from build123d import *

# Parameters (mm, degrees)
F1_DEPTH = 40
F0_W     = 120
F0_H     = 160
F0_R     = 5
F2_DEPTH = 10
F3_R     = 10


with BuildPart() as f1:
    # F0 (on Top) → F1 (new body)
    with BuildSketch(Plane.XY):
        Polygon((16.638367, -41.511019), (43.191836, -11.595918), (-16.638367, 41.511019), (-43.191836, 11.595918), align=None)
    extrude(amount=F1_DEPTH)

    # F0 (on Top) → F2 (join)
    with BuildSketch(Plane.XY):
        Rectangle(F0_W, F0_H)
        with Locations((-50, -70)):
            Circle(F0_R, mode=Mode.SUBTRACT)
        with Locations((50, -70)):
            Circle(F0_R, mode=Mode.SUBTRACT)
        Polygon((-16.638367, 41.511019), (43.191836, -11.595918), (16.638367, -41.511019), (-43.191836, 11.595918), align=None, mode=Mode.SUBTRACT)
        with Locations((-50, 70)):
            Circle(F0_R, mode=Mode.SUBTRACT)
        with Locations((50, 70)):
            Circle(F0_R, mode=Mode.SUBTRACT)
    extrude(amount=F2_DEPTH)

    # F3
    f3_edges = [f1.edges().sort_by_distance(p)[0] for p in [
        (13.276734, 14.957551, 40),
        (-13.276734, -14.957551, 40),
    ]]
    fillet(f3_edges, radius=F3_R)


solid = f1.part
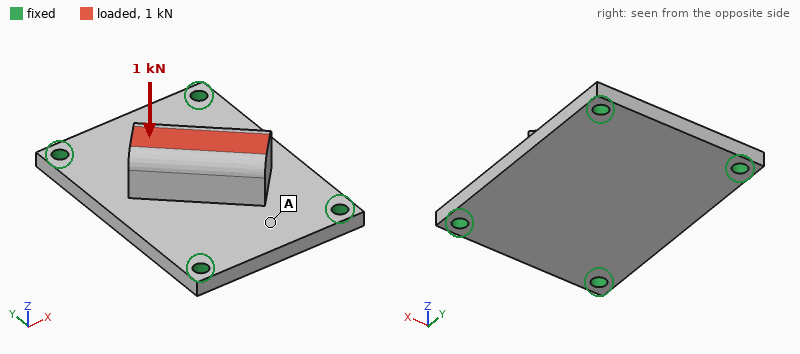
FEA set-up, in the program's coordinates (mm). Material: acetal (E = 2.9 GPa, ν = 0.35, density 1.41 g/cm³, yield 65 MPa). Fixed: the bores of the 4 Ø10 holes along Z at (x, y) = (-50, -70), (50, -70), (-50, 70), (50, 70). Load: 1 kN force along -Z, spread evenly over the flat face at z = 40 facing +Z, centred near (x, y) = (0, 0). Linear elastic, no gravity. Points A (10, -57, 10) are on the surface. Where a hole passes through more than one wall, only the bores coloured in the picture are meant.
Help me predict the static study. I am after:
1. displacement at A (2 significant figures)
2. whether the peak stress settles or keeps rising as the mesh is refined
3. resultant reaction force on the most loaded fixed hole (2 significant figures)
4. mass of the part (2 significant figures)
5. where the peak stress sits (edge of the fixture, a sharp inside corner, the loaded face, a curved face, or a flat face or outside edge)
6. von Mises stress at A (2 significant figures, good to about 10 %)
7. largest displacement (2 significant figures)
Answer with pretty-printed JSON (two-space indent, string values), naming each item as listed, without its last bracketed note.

{
  "displacement at A": "0.18 mm",
  "whether the peak stress settles or keeps rising as the mesh is refined": "keeps rising",
  "resultant reaction force on the most loaded fixed hole": "350 N",
  "mass of the part": "400 g",
  "where the peak stress sits": "edge of the fixture",
  "von Mises stress at A": "2.7 MPa",
  "largest displacement": "0.33 mm"
}
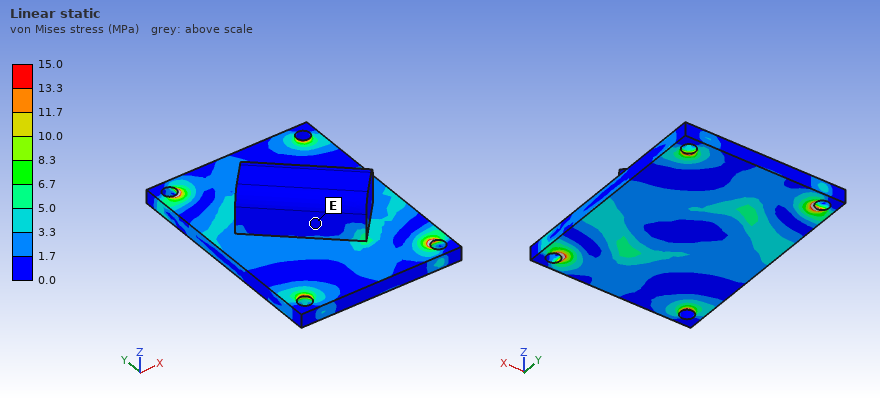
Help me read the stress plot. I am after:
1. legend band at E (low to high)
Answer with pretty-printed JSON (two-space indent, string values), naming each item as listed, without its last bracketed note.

{
  "legend band at E": "0.0 to 1.7 MPa"
}
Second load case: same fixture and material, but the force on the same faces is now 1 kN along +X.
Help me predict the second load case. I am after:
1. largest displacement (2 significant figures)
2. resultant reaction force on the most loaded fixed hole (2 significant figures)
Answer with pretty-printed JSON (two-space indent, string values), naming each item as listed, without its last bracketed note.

{
  "largest displacement": "0.41 mm",
  "resultant reaction force on the most loaded fixed hole": "360 N"
}
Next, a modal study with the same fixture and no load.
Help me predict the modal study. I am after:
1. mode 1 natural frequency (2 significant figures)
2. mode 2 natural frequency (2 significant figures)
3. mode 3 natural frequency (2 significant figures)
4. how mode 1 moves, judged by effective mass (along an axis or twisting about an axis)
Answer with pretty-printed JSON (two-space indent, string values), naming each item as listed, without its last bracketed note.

{
  "mode 1 natural frequency": "550 Hz",
  "mode 2 natural frequency": "740 Hz",
  "mode 3 natural frequency": "1100 Hz",
  "how mode 1 moves, judged by effective mass": "along Z"
}
